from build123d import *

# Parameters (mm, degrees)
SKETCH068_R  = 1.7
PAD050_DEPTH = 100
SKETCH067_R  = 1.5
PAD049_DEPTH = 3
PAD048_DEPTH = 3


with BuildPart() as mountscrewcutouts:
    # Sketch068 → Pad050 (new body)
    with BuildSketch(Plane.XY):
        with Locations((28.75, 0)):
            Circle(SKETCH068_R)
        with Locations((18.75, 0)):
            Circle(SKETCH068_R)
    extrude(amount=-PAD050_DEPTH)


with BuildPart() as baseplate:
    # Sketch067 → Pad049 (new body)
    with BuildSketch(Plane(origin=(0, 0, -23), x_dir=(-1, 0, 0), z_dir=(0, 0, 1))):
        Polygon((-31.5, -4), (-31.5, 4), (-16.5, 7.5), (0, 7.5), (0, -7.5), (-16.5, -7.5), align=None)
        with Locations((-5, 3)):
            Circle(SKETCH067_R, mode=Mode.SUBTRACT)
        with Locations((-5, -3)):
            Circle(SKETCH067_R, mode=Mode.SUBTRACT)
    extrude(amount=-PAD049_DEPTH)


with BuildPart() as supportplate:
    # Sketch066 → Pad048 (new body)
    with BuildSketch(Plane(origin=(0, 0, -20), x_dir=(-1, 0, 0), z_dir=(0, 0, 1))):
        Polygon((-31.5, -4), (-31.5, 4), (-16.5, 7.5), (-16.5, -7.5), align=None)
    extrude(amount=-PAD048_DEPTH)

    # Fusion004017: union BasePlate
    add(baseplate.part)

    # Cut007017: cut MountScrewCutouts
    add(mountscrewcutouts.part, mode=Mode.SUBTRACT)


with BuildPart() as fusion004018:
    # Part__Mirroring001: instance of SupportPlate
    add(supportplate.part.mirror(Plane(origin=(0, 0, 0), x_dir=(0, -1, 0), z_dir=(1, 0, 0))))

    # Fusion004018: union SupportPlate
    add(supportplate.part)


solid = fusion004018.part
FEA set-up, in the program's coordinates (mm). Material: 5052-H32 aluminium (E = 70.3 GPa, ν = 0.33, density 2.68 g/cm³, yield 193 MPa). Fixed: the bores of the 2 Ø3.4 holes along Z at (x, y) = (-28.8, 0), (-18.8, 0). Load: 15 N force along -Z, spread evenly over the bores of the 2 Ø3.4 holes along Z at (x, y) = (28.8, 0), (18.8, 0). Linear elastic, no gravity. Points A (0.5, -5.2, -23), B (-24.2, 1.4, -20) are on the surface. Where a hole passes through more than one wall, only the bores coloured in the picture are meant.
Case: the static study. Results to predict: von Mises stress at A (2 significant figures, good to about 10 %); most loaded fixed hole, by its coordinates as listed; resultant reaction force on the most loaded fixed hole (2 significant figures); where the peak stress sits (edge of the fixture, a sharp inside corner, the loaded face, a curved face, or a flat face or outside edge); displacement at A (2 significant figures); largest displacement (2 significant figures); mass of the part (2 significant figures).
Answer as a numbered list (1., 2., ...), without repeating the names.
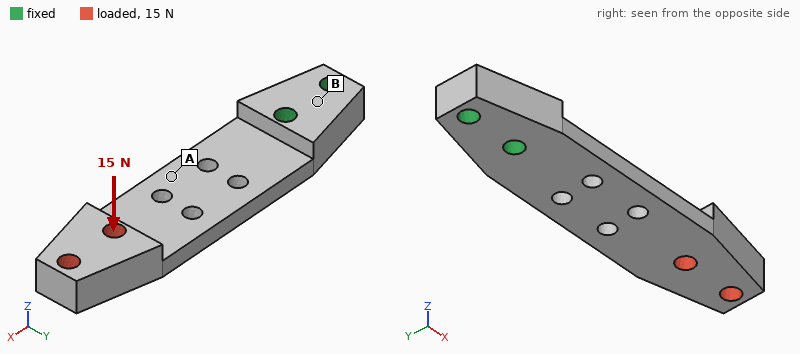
1. 16 MPa
2. (-18.8, 0)
3. 32 N
4. a curved face
5. 0.039 mm
6. 0.21 mm
7. 8.7 g
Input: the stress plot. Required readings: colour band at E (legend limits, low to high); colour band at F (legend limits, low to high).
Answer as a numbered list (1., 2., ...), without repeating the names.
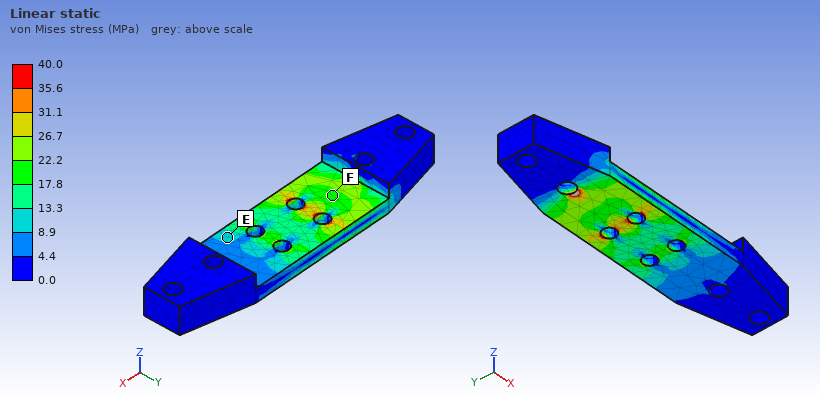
1. 8.9 to 13.3 MPa
2. 17.8 to 22.2 MPa
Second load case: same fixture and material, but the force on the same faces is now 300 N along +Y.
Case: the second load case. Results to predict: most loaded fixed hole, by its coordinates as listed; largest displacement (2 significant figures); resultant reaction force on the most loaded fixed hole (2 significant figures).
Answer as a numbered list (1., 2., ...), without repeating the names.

1. (-18.8, 0)
2. 0.27 mm
3. 1.1 kN
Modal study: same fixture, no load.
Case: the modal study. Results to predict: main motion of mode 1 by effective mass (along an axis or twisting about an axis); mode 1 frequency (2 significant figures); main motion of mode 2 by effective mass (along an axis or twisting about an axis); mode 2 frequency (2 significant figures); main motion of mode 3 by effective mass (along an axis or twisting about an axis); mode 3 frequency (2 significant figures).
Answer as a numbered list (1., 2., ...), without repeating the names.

1. along Z
2. 880 Hz
3. along Y
4. 3400 Hz
5. twisting about X
6. 5900 Hz
